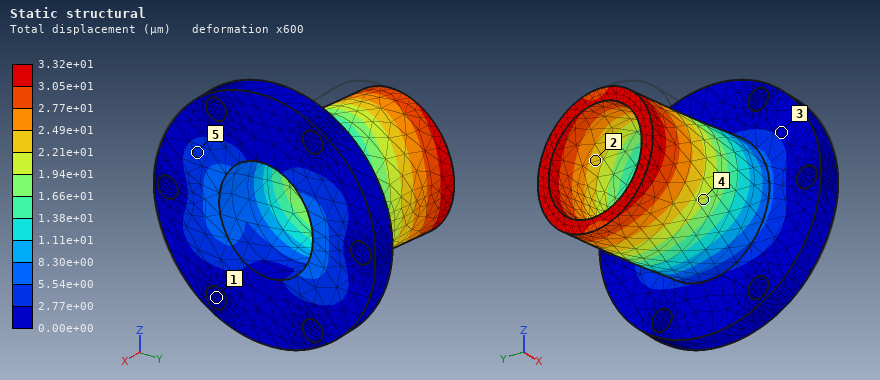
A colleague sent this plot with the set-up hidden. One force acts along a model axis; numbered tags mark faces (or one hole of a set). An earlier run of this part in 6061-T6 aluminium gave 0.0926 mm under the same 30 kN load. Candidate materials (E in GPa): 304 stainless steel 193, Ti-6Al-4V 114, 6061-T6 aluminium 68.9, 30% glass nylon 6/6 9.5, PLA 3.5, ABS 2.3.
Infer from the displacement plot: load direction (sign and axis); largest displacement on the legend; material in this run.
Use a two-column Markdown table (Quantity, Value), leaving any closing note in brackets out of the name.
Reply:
| Quantity | Value |
|---|---|
| load direction | +Y |
| largest displacement on the legend | 3.32e+01 µm |
| material in this run | 304 stainless steel |
